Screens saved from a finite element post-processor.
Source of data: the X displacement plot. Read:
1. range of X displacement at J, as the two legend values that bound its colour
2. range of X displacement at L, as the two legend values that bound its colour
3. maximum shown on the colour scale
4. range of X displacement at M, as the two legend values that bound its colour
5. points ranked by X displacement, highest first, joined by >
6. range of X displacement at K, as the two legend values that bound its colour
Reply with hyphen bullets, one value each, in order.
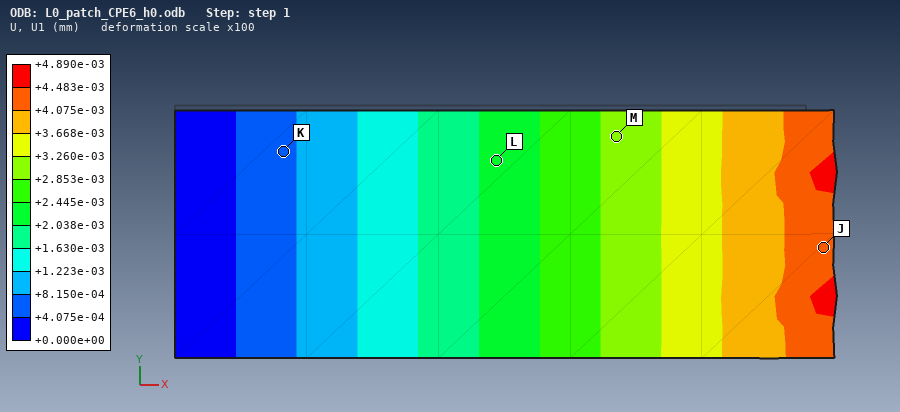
- +4.075e-03 to +4.483e-03 mm
- +2.038e-03 to +2.445e-03 mm
- +4.890e-03 mm
- +2.853e-03 to +3.260e-03 mm
- J > M > L > K
- +4.075e-04 to +8.150e-04 mm
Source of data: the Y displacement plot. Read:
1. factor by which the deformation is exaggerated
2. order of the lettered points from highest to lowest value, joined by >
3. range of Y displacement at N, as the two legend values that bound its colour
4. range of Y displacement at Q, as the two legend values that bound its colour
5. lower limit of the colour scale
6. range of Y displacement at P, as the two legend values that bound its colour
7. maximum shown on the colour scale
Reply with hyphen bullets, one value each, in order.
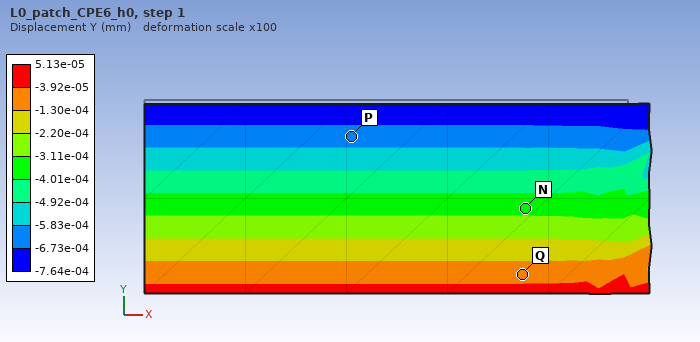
- 100
- Q > N > P
- -4.01e-04 to -3.11e-04 mm
- -1.30e-04 to -3.92e-05 mm
- -7.64e-04 mm
- -6.73e-04 to -5.83e-04 mm
- 5.13e-05 mm
